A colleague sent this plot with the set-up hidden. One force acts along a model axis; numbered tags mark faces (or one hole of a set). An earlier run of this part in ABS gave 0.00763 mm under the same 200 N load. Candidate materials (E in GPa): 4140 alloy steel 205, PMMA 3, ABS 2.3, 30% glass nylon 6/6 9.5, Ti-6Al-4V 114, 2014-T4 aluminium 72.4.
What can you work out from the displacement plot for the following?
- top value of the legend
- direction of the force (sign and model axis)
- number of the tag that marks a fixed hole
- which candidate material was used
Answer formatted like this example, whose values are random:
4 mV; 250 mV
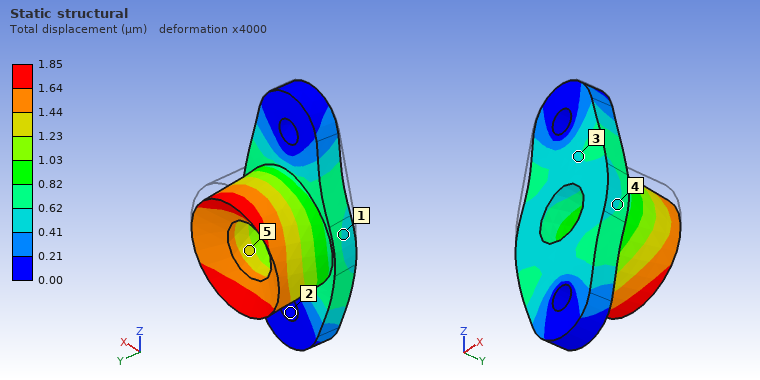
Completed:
1.85 µm; -Z; 2; 30% glass nylon 6/6
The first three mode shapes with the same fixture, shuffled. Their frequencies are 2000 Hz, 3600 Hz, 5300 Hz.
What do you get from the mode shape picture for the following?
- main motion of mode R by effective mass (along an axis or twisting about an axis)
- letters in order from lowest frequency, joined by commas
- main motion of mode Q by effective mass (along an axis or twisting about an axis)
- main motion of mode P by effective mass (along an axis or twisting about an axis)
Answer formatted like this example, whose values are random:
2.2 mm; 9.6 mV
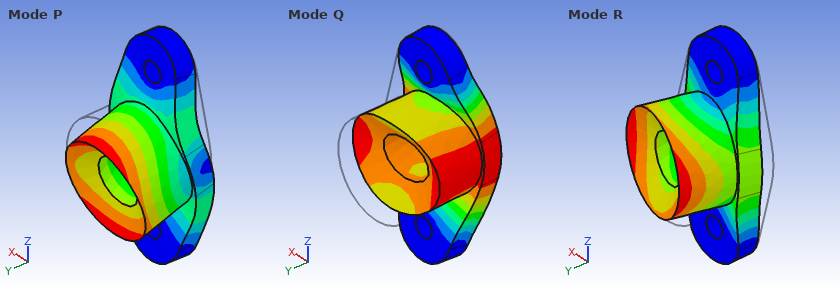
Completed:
along X; R, Q, P; along Y; along Z
